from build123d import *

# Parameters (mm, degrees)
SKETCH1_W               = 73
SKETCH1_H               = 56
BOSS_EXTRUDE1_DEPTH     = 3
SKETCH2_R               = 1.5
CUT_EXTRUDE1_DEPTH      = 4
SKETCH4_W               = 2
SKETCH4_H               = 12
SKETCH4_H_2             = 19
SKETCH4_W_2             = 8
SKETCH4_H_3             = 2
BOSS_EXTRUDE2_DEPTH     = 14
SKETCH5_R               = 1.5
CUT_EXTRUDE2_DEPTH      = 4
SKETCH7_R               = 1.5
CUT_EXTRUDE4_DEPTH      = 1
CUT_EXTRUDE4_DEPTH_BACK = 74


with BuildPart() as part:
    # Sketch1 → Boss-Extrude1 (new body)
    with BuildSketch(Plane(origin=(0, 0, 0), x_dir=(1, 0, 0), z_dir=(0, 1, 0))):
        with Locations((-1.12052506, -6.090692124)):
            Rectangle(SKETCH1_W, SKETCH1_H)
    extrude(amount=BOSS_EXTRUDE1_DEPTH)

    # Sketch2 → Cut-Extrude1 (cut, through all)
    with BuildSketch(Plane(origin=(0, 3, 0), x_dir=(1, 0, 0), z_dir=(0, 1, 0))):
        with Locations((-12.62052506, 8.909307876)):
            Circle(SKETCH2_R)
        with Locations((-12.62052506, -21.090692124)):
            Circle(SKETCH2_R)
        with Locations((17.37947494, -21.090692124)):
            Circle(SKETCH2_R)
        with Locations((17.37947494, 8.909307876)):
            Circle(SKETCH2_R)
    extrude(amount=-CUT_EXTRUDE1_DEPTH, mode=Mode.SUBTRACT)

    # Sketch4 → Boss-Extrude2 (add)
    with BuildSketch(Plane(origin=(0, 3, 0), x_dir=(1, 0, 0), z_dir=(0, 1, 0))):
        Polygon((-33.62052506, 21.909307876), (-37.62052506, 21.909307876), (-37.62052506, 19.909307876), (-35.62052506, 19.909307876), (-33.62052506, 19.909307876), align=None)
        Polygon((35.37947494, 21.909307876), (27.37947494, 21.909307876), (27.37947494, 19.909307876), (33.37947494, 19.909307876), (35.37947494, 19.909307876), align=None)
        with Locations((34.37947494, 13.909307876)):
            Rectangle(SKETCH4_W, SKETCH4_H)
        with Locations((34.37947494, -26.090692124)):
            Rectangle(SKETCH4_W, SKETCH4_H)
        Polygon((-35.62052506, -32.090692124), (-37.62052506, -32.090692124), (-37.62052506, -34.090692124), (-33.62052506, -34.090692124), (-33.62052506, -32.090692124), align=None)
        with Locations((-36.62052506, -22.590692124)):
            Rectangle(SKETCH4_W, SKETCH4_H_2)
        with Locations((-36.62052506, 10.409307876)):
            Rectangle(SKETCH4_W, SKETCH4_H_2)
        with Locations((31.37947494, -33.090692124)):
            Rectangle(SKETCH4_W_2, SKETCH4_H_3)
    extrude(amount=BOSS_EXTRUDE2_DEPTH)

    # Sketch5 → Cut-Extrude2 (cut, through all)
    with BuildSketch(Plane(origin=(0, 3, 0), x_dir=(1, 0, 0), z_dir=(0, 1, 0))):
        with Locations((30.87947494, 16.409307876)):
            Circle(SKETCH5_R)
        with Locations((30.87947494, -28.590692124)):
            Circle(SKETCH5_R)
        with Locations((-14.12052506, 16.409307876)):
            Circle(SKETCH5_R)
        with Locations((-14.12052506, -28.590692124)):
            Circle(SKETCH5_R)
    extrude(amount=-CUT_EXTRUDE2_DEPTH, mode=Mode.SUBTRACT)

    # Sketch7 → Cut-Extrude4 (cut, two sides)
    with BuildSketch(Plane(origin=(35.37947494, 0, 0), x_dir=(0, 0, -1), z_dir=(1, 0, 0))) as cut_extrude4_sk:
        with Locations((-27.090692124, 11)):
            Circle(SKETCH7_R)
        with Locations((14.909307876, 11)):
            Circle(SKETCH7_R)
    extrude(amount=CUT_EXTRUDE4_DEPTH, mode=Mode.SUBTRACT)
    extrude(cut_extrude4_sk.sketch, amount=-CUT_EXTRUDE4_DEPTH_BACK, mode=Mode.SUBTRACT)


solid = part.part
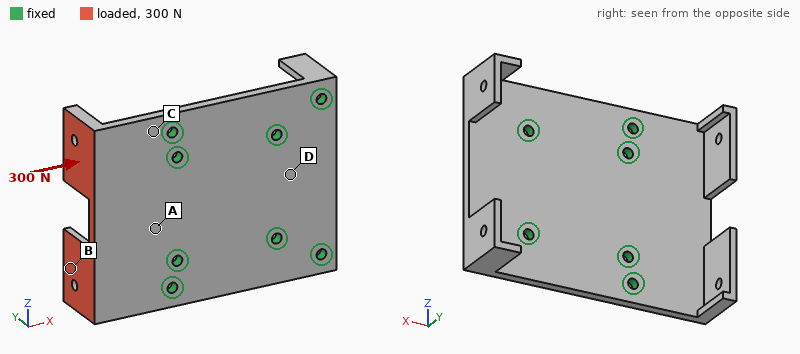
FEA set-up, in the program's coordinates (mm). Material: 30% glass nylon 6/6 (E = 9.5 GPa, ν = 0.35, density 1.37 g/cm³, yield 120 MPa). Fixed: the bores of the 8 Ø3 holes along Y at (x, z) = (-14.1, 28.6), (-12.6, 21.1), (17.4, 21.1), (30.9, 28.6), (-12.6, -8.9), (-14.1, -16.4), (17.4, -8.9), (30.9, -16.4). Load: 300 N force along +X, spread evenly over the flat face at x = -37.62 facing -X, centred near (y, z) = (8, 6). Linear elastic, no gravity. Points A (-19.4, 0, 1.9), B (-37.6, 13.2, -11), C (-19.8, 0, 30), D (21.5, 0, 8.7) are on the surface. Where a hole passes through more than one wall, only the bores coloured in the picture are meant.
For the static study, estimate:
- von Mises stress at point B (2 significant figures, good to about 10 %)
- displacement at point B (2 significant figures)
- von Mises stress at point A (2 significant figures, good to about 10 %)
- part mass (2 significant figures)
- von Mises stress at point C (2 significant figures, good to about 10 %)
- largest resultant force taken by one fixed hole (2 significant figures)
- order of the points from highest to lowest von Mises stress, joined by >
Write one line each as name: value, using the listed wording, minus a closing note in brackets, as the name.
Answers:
von Mises stress at point B: 7.7 MPa
displacement at point B: 0.79 mm
von Mises stress at point A: 17 MPa
part mass: 20 g
von Mises stress at point C: 24 MPa
largest resultant force taken by one fixed hole: 69 N
order of the points from highest to lowest von Mises stress, joined by >: C > A > B > D
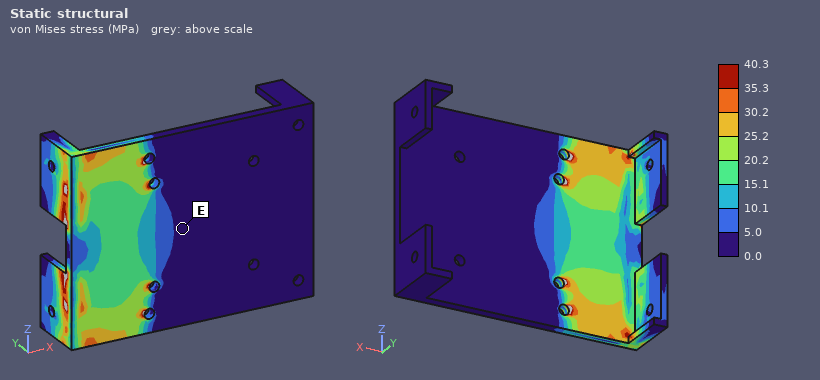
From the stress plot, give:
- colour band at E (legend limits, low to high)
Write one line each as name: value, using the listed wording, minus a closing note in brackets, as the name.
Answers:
colour band at E: 0.0 to 5.0 MPa
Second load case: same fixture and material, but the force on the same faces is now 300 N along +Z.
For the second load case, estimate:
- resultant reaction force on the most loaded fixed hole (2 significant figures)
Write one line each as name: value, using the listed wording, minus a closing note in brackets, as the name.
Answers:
resultant reaction force on the most loaded fixed hole: 150 N
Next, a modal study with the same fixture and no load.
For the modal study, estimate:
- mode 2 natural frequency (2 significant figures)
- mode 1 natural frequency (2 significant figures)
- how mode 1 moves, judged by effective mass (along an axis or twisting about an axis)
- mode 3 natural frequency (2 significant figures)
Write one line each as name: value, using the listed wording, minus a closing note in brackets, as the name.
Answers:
mode 2 natural frequency: 1800 Hz
mode 1 natural frequency: 1400 Hz
how mode 1 moves, judged by effective mass: along Y
mode 3 natural frequency: 2900 Hz
